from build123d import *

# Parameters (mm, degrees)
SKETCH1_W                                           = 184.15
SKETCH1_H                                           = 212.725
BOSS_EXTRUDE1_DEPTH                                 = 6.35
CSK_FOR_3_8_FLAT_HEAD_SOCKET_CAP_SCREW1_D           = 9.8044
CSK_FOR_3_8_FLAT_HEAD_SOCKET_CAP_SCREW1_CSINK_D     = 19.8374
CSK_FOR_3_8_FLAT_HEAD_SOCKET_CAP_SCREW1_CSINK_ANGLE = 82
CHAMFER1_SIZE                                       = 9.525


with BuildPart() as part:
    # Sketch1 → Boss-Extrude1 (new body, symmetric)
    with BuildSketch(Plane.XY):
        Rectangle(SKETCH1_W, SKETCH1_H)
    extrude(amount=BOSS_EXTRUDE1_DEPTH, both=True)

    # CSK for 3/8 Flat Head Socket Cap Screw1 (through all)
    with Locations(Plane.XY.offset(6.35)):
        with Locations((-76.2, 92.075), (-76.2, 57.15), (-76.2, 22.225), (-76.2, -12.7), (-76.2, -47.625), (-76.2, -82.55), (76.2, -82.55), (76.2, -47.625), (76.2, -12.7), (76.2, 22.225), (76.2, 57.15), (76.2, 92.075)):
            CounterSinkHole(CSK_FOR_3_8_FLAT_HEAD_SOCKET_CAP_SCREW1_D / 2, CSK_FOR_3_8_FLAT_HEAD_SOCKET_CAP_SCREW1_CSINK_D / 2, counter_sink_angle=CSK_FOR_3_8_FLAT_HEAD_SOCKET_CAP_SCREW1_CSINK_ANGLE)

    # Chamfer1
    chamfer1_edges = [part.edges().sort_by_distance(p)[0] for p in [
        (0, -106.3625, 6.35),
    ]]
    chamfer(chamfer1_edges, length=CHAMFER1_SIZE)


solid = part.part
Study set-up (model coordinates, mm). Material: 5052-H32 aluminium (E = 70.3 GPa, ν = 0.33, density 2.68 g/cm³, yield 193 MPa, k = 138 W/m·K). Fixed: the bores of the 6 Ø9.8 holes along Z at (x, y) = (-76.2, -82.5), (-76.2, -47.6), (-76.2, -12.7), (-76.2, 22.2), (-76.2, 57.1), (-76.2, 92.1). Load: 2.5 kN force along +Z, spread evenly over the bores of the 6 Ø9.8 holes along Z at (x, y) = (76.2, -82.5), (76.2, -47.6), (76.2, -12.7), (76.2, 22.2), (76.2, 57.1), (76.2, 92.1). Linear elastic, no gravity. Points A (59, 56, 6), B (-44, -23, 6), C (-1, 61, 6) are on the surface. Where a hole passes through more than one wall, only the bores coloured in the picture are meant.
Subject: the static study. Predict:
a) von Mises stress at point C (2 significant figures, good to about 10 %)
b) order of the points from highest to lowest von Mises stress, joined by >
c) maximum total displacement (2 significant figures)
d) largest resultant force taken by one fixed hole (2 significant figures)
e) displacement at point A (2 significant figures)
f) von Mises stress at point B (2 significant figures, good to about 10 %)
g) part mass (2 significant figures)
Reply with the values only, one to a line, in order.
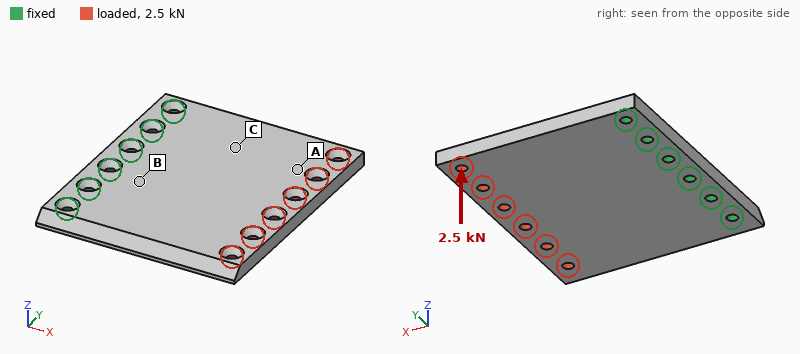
32 MPa
B > C > A
1.5 mm
890 N
1.1 mm
48 MPa
1.3 kg
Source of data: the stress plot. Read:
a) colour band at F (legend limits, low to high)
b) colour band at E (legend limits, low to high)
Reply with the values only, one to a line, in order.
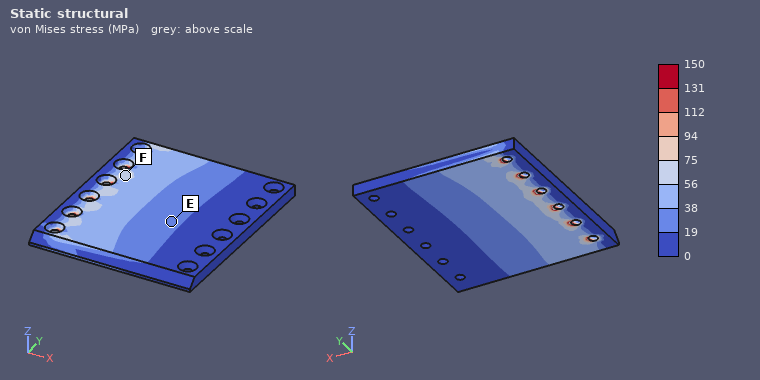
56 to 75 MPa
19 to 38 MPa
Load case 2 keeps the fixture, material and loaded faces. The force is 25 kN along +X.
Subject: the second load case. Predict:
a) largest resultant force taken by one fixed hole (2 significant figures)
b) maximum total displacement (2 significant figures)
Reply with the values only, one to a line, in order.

4.7 kN
0.37 mm
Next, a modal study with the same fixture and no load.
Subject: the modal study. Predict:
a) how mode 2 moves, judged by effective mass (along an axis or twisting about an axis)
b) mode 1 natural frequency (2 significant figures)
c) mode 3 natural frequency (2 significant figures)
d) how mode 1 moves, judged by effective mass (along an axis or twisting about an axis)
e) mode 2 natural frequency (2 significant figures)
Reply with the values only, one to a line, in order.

twisting about X
350 Hz
1900 Hz
along Z
740 Hz
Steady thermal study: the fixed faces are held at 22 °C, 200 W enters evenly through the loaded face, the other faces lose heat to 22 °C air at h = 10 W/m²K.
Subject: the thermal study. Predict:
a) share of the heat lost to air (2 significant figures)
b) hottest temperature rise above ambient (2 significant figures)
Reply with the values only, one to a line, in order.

16 %
83 K
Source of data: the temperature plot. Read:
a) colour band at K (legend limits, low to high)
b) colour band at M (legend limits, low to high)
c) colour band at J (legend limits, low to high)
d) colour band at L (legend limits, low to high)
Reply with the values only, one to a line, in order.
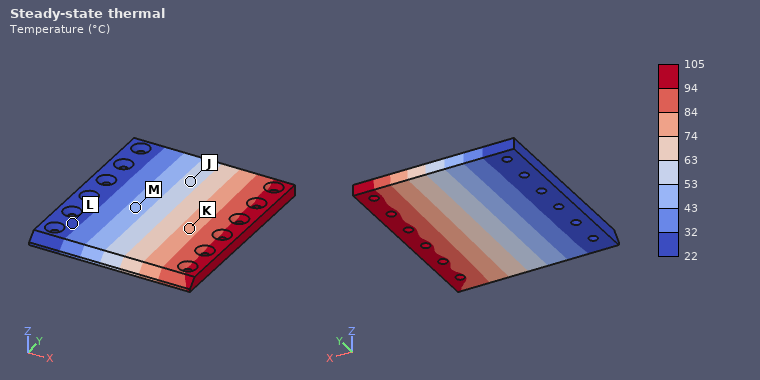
74 to 84 °C
43 to 53 °C
53 to 63 °C
22 to 32 °C
